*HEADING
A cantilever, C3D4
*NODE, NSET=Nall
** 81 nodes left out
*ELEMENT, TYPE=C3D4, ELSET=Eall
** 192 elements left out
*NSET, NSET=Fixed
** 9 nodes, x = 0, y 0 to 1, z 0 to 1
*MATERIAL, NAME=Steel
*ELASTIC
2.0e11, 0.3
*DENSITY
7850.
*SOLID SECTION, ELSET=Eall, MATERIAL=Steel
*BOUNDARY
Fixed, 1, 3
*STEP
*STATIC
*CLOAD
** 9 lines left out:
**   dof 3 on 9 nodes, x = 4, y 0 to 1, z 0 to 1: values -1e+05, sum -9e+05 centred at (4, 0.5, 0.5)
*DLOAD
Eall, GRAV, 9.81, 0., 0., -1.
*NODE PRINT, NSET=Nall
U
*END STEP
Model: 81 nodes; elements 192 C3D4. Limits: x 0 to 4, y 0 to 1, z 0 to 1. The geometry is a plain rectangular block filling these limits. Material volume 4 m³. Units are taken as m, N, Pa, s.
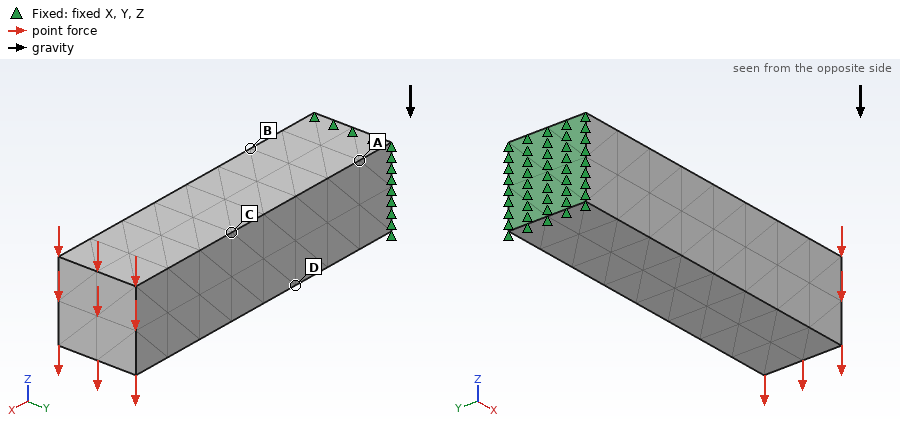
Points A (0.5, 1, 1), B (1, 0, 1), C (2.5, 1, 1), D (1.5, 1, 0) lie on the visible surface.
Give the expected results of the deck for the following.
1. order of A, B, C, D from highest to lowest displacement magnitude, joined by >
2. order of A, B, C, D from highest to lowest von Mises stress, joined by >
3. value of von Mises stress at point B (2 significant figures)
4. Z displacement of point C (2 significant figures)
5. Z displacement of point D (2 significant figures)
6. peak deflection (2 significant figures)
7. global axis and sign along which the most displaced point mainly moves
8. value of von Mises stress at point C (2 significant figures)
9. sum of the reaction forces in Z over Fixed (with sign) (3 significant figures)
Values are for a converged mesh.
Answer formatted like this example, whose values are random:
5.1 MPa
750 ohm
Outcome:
C > D > B > A
A > B > D > C
1.8e+07 Pa
-6.4e-04 m
-2.6e-04 m
0.0014 m
-Z
8.7e+06 Pa
1.21e+06 N
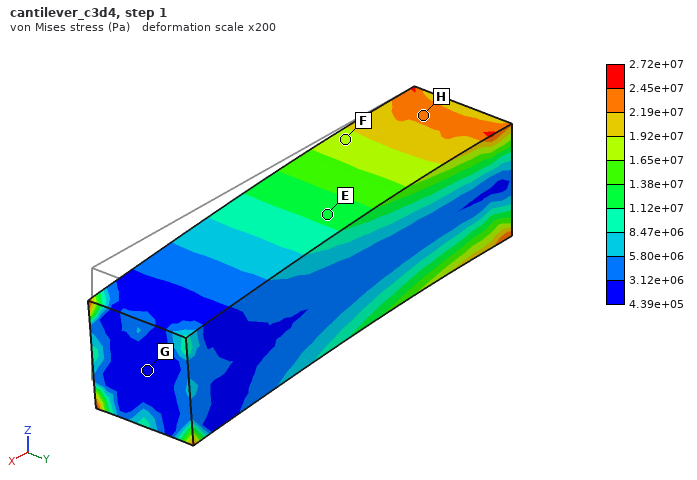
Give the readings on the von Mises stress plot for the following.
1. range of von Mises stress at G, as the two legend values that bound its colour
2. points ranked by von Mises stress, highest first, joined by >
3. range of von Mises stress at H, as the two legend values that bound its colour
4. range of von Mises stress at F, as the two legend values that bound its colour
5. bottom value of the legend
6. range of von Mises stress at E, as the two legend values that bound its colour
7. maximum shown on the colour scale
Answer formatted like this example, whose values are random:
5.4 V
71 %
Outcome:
4.39e+05 to 3.12e+06 Pa
H > F > E > G
2.19e+07 to 2.45e+07 Pa
1.65e+07 to 1.92e+07 Pa
4.39e+05 Pa
1.12e+07 to 1.38e+07 Pa
2.72e+07 Pa
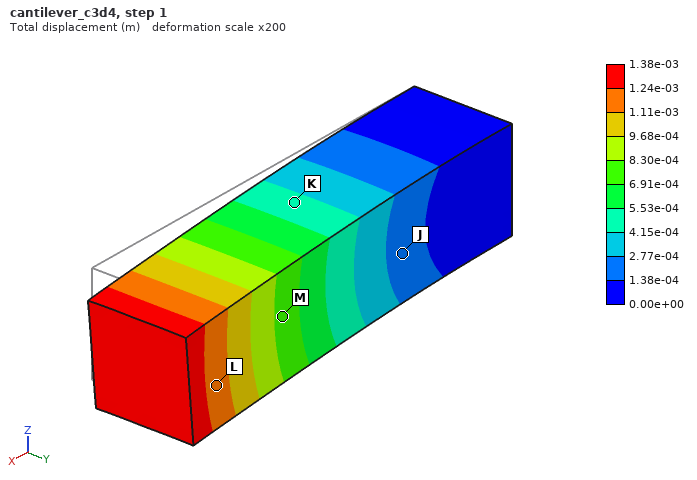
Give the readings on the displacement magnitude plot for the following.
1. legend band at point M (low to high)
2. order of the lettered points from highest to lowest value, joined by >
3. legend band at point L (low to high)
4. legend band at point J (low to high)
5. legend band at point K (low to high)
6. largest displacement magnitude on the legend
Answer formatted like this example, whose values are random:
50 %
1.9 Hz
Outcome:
6.91e-04 to 8.30e-04 m
L > M > K > J
1.11e-03 to 1.24e-03 m
1.38e-04 to 2.77e-04 m
4.15e-04 to 5.53e-04 m
1.38e-03 m
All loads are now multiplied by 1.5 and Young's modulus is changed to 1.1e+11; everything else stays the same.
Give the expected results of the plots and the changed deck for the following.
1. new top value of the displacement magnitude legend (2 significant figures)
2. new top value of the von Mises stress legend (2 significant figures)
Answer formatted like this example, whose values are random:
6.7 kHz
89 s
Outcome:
0.0038 m
4.1e+07 Pa
